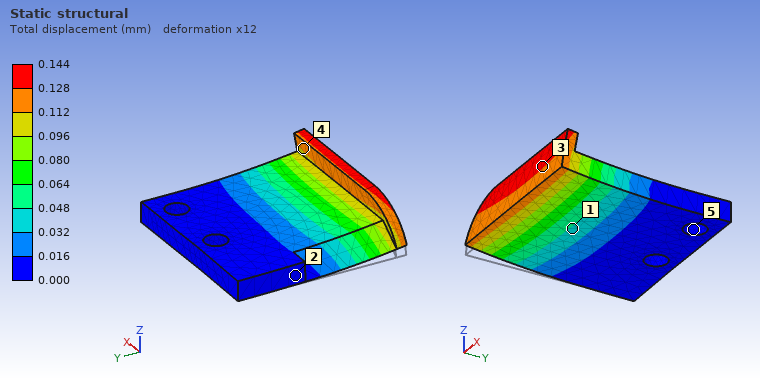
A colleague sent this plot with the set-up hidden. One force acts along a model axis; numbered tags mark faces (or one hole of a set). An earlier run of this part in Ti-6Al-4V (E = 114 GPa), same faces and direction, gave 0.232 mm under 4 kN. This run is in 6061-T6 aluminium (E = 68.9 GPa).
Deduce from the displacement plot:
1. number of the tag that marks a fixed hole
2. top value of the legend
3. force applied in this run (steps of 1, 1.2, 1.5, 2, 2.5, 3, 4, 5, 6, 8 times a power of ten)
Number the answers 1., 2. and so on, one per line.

1. 5
2. 0.144 mm
3. 1.5 kN
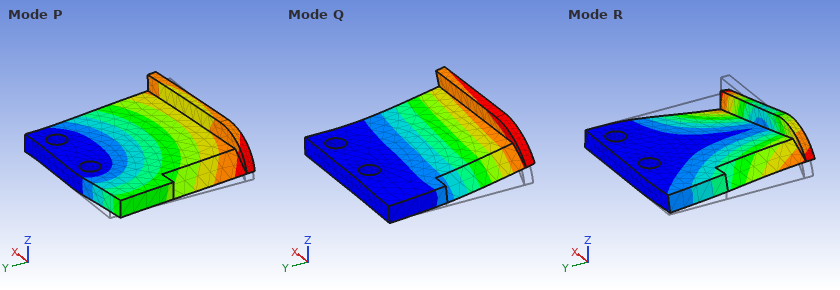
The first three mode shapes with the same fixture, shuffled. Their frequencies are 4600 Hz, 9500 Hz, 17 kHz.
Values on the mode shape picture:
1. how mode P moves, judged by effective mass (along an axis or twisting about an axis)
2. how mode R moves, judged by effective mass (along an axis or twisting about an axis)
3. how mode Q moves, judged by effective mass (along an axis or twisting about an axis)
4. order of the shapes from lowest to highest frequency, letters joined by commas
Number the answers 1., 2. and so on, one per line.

1. along X
2. twisting about Y
3. along Z
4. Q, R, P
